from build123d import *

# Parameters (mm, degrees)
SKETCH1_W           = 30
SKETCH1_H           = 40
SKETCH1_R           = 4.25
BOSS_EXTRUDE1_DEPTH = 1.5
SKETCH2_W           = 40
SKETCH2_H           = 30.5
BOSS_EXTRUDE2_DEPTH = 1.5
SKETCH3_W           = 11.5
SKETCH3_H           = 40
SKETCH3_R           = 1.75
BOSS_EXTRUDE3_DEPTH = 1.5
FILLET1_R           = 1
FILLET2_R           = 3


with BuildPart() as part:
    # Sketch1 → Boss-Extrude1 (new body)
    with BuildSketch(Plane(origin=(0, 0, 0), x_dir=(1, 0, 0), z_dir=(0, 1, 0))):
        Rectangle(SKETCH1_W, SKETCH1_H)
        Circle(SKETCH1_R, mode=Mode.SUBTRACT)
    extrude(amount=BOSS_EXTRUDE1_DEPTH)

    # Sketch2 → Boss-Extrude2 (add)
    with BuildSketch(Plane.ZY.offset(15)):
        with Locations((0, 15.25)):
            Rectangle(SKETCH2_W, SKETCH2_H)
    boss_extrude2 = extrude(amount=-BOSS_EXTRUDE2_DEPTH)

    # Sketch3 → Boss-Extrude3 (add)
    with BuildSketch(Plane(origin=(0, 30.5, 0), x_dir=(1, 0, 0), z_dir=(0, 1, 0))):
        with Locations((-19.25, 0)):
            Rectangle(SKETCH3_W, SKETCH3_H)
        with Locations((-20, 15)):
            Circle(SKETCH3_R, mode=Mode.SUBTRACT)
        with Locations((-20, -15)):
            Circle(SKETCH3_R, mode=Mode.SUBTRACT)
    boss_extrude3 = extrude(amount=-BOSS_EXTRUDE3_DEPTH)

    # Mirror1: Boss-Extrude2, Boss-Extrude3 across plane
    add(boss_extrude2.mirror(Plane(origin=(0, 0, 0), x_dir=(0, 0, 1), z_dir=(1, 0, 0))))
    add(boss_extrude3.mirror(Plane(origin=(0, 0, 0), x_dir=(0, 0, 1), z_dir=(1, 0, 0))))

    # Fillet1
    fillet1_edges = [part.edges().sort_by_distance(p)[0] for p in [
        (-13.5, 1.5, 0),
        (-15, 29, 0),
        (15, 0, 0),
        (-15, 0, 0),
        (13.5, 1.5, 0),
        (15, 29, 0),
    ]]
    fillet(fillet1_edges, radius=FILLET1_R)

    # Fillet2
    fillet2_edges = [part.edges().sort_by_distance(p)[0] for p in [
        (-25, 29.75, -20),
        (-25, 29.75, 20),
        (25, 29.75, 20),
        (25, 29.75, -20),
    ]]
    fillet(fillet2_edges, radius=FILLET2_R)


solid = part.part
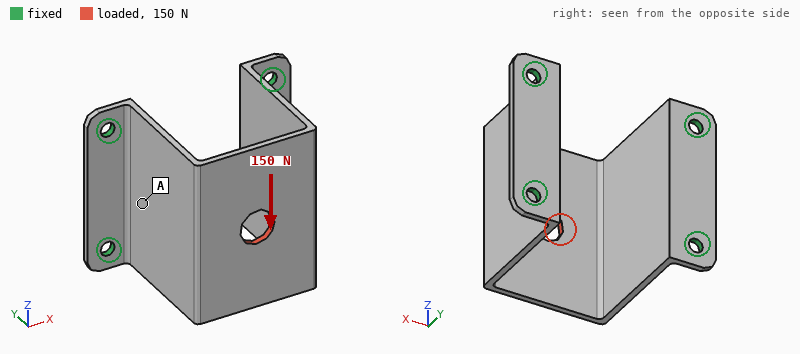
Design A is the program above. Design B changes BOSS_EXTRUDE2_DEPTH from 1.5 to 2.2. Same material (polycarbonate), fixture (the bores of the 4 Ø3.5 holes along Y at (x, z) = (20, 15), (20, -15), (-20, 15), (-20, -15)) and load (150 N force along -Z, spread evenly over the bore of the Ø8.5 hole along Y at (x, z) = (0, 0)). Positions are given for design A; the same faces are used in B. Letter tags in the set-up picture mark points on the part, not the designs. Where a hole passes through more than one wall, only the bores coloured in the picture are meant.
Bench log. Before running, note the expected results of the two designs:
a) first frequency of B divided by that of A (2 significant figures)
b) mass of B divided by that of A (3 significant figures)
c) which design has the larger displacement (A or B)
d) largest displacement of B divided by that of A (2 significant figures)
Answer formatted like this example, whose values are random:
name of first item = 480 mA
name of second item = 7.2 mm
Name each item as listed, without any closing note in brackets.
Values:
first frequency of B divided by that of A = 1.2
mass of B divided by that of A = 1.26
which design has the larger displacement = A
largest displacement of B divided by that of A = 0.80
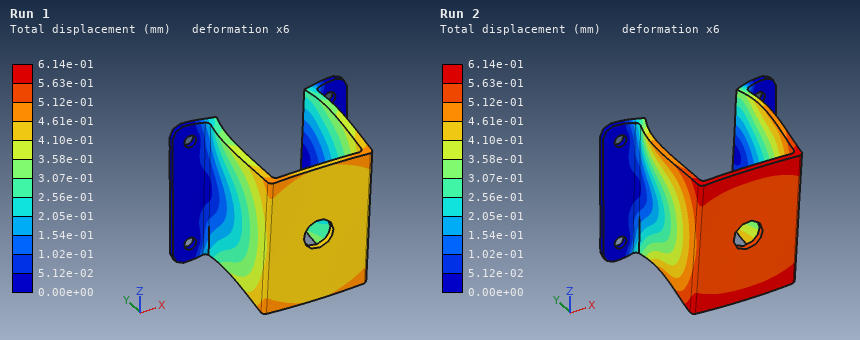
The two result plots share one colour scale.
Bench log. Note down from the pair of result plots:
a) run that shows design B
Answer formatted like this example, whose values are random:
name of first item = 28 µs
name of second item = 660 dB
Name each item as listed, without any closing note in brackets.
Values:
run that shows design B = Run 1
